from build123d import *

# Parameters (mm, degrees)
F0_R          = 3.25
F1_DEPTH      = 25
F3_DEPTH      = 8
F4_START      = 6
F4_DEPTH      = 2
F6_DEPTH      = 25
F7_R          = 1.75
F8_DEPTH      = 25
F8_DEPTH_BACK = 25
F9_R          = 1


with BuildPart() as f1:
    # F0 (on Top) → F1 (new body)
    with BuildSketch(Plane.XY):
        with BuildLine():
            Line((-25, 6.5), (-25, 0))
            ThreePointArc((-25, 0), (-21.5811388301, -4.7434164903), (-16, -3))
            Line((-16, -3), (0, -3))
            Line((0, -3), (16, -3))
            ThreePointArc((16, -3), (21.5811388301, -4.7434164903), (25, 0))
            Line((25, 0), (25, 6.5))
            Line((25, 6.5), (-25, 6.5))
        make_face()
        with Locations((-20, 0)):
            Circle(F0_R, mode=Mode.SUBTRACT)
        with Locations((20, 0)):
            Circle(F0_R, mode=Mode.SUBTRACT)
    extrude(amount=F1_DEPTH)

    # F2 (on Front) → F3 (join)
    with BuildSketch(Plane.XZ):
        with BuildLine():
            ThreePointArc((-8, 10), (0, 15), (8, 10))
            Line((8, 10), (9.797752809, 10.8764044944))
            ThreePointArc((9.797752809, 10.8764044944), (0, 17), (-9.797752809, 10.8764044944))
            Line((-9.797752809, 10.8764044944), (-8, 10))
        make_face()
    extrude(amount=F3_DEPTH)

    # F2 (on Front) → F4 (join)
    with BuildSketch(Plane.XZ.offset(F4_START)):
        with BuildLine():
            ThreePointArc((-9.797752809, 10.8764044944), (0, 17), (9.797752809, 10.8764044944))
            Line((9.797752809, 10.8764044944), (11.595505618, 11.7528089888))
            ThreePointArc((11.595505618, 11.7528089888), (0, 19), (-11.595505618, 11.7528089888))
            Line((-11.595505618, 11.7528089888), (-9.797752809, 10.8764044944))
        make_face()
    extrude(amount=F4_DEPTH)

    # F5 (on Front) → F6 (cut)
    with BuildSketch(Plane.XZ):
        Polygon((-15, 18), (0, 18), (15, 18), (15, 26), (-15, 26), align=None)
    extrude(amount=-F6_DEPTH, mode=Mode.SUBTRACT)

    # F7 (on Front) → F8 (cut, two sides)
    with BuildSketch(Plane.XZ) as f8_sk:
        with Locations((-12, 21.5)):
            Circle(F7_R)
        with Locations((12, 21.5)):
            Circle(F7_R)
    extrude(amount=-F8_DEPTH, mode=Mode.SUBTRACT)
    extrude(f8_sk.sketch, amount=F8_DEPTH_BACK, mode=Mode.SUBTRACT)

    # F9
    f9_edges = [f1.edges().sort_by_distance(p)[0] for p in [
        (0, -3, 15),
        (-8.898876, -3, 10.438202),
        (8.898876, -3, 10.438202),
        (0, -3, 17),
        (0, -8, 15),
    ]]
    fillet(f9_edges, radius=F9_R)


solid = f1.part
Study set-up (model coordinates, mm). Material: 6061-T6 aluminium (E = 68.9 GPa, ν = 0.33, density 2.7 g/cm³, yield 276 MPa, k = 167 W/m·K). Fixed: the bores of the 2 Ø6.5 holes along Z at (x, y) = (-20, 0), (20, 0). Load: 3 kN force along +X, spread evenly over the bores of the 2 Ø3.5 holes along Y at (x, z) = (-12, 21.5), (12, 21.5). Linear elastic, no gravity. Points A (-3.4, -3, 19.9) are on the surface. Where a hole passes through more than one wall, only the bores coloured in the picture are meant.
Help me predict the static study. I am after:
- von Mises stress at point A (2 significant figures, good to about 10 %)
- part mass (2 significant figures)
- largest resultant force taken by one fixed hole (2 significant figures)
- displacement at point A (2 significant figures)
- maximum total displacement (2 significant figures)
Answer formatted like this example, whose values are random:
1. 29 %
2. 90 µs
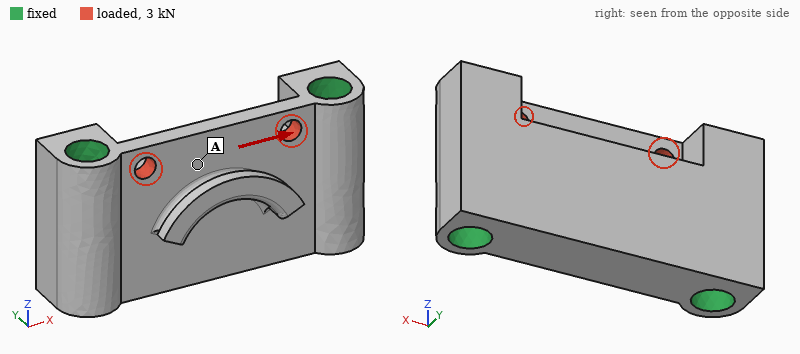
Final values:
1. 13 MPa
2. 26 g
3. 1.5 kN
4. 2.4 µm
5. 5.6 µm
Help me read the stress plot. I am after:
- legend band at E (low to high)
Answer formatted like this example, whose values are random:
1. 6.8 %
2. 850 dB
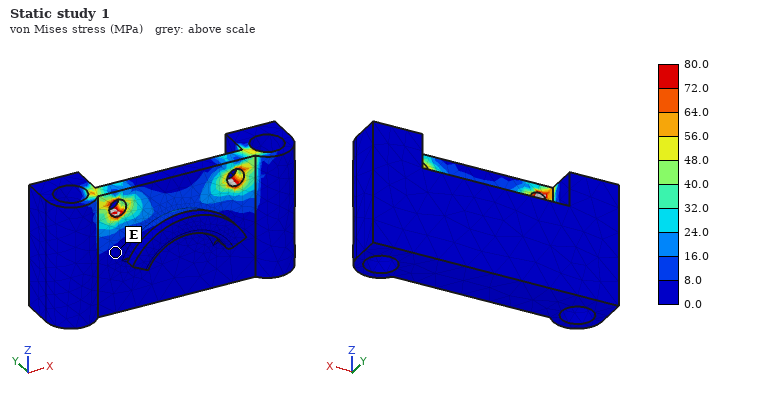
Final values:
1. 0.0 to 8.0 MPa
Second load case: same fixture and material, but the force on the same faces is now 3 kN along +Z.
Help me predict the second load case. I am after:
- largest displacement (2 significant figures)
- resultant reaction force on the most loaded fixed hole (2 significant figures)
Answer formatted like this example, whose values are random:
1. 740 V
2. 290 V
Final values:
1. 9.7 µm
2. 1.5 kN
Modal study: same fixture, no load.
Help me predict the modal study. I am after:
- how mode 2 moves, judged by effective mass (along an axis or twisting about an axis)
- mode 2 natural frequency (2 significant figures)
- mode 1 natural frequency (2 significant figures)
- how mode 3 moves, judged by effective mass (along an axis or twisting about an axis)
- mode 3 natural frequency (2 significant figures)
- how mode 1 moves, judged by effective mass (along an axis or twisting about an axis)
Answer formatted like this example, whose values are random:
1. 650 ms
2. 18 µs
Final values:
1. along Y
2. 30 kHz
3. 24 kHz
4. along Z
5. 36 kHz
6. along Y
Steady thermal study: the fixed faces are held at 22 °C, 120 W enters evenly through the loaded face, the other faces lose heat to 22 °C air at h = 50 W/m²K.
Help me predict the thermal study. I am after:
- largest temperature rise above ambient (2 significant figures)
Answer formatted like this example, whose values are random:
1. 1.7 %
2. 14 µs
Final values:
1. 53 K
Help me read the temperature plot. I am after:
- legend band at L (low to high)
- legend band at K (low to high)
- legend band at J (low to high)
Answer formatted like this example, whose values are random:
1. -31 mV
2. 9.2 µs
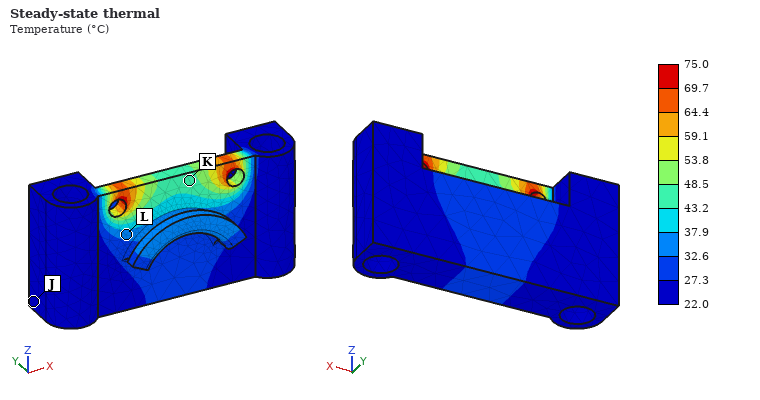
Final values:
1. 32.6 to 37.9 °C
2. 43.2 to 48.5 °C
3. 22.0 to 27.3 °C
